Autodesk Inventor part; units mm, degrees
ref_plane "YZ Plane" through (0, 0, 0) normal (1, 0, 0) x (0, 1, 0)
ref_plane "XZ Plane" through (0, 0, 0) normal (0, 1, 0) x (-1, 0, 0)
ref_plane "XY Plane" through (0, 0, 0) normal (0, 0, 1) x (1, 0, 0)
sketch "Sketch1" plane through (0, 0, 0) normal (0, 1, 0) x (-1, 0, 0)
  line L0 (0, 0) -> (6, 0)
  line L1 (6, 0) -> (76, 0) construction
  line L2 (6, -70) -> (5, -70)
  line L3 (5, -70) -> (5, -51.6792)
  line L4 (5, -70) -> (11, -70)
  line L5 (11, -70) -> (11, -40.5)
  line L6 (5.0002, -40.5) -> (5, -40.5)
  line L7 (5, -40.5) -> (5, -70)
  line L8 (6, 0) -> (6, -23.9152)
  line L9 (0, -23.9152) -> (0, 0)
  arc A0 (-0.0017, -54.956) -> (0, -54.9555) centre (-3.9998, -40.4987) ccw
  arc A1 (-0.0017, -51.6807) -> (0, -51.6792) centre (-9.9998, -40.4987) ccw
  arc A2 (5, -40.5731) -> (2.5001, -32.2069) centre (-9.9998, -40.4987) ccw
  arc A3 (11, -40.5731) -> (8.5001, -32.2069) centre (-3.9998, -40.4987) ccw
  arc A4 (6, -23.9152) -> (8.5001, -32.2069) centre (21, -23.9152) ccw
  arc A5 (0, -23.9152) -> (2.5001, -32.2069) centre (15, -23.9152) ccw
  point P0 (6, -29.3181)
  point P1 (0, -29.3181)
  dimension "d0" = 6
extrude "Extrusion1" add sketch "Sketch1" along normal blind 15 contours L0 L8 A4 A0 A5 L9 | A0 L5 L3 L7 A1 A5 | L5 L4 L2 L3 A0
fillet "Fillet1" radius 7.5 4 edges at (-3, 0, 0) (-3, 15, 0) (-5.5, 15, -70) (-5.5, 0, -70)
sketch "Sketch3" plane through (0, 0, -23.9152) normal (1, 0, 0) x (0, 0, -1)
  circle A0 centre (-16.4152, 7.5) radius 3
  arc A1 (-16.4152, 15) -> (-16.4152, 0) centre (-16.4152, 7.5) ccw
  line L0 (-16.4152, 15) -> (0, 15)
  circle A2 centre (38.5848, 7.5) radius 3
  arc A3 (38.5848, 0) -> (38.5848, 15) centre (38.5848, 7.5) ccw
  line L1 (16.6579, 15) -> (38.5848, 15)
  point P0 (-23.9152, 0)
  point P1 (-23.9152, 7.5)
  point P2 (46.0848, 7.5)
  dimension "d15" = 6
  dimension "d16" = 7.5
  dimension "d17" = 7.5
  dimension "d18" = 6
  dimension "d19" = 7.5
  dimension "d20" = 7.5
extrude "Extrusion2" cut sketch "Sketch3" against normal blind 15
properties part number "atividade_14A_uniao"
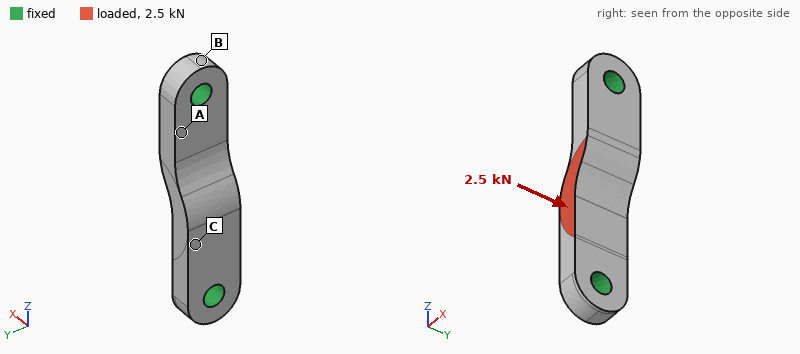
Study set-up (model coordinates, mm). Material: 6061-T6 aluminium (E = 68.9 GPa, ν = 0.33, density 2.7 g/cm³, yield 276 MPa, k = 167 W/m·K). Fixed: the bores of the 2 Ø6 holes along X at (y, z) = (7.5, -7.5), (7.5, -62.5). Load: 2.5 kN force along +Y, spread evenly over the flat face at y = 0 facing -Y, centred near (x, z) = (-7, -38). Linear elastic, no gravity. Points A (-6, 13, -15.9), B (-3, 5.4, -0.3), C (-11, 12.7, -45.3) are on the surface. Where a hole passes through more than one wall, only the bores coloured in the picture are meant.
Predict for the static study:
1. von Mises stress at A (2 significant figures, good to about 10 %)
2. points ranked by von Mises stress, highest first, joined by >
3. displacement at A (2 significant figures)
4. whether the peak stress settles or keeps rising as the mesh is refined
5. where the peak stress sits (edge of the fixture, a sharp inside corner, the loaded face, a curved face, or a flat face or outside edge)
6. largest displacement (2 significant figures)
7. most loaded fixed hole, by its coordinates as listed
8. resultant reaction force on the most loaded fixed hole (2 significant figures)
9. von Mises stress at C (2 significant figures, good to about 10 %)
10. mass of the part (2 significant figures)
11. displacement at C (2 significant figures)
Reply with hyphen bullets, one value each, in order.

- 22 MPa
- C > A > B
- 11 µm
- keeps rising
- edge of the fixture
- 45 µm
- (7.5, -62.5)
- 1.5 kN
- 34 MPa
- 15 g
- 32 µm
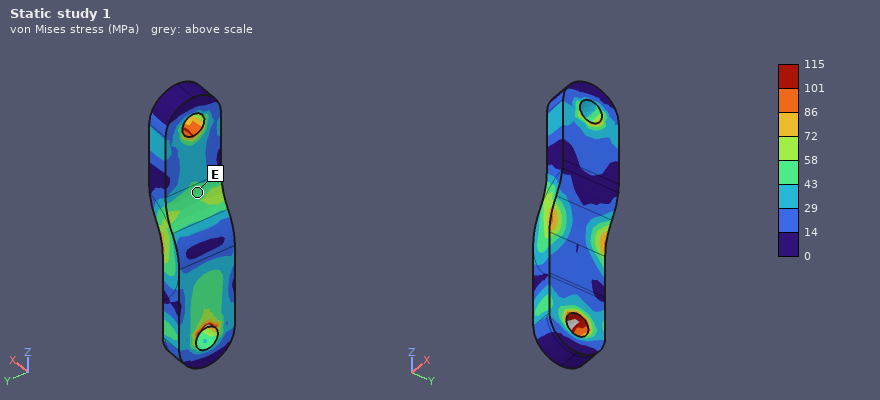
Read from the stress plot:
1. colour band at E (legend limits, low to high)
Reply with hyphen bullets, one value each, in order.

- 43 to 58 MPa
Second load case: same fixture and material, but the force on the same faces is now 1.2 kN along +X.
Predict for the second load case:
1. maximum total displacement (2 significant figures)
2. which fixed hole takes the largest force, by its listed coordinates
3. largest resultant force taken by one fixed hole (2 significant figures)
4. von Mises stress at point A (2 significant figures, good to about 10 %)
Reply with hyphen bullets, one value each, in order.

- 83 µm
- (7.5, -62.5)
- 780 N
- 32 MPa
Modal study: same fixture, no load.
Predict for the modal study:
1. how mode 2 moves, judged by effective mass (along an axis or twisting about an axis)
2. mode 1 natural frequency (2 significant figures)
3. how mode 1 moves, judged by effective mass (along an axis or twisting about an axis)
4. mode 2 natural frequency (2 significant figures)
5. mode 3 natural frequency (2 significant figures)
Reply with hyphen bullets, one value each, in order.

- along Y
- 10 kHz
- along X
- 16 kHz
- 20 kHz
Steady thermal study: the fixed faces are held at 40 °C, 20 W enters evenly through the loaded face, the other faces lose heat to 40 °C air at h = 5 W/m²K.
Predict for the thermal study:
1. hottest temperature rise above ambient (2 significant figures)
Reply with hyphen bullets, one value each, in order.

- 18 K
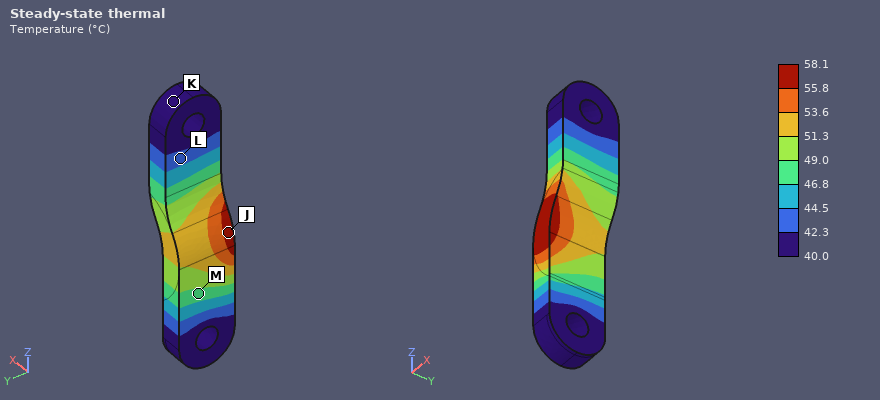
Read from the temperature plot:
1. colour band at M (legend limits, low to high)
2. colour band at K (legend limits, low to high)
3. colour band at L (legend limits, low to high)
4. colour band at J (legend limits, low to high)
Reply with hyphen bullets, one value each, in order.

- 46.8 to 49.0 °C
- 40.0 to 42.3 °C
- 42.3 to 44.5 °C
- 55.8 to 58.1 °C
